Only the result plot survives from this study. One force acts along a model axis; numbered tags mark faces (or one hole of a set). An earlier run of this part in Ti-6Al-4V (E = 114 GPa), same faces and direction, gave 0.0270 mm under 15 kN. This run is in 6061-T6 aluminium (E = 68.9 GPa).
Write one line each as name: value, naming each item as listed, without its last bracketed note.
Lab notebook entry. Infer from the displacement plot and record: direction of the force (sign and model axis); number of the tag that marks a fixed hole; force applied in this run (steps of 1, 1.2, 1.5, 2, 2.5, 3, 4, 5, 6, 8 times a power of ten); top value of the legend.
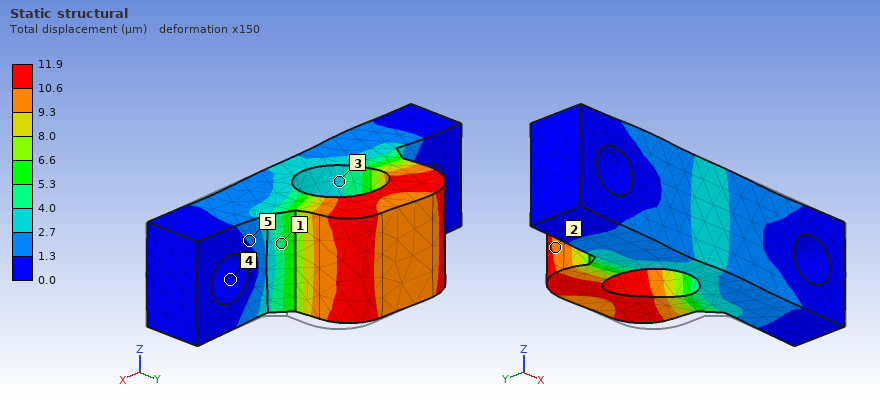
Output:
direction of the force: -X
number of the tag that marks a fixed hole: 4
force applied in this run: 4 kN
top value of the legend: 11.9 µm
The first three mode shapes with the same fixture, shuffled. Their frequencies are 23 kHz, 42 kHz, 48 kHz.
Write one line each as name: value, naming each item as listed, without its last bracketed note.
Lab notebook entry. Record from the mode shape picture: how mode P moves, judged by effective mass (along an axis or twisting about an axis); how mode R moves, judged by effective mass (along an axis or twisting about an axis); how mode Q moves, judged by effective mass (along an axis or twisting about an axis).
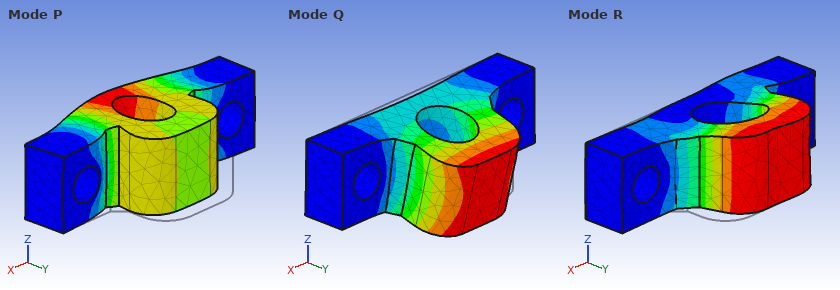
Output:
how mode P moves, judged by effective mass: along Y
how mode R moves, judged by effective mass: along X
how mode Q moves, judged by effective mass: along Z
